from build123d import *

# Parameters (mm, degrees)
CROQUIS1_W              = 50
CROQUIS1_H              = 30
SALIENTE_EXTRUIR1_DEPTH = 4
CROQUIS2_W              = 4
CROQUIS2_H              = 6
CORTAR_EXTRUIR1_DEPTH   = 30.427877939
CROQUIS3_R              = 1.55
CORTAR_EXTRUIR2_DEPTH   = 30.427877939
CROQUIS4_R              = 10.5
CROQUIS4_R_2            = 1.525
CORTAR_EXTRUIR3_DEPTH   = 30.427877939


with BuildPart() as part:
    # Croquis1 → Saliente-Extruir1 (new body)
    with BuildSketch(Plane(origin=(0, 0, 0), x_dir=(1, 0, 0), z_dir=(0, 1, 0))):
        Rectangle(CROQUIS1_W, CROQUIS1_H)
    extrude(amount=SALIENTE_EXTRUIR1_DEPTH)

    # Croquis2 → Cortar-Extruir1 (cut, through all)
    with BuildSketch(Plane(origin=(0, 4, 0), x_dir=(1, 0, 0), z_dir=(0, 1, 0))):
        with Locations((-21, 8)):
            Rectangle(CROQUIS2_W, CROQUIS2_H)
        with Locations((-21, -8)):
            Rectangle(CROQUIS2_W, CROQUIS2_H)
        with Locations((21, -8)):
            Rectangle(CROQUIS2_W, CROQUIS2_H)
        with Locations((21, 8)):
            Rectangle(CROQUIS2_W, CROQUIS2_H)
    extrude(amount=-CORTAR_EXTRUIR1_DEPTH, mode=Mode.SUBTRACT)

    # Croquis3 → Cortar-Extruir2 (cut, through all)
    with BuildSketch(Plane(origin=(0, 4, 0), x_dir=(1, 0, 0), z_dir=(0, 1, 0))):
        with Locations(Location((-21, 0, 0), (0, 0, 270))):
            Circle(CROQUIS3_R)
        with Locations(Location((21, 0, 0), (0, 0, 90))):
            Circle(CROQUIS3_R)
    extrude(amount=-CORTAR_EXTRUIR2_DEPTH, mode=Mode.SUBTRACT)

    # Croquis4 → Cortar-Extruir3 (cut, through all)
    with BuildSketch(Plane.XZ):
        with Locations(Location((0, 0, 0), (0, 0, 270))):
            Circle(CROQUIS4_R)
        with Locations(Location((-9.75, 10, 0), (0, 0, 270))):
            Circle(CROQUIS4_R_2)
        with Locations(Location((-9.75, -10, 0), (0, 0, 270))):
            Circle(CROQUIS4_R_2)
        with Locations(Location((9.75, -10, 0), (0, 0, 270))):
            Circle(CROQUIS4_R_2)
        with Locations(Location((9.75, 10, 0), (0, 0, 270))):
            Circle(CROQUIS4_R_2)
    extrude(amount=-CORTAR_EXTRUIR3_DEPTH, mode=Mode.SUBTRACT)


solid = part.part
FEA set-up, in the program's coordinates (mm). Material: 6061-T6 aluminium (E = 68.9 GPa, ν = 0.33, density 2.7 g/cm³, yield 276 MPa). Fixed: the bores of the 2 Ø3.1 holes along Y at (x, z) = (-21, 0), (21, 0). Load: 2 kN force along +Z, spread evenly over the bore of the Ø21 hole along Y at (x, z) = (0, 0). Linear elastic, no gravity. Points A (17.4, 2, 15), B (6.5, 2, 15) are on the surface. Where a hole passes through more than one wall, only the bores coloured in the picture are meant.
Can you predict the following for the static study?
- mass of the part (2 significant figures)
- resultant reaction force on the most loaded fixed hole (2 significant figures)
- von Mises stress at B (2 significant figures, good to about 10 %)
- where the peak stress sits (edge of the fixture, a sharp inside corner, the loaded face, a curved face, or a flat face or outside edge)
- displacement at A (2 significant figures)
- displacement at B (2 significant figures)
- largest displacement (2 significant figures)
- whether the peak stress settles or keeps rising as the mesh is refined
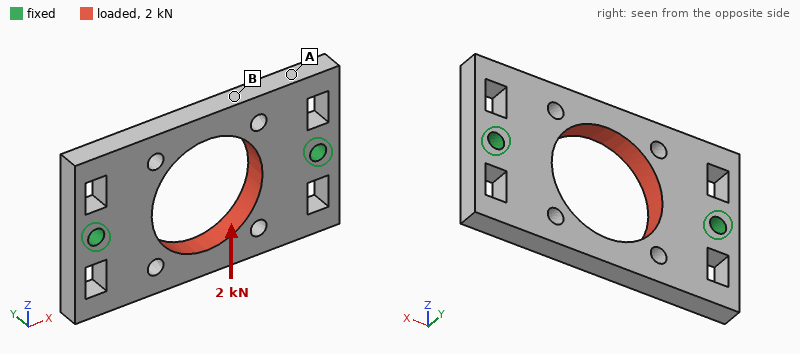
11 g
1.0 kN
29 MPa
edge of the fixture
6.9 µm
12 µm
15 µm
keeps rising
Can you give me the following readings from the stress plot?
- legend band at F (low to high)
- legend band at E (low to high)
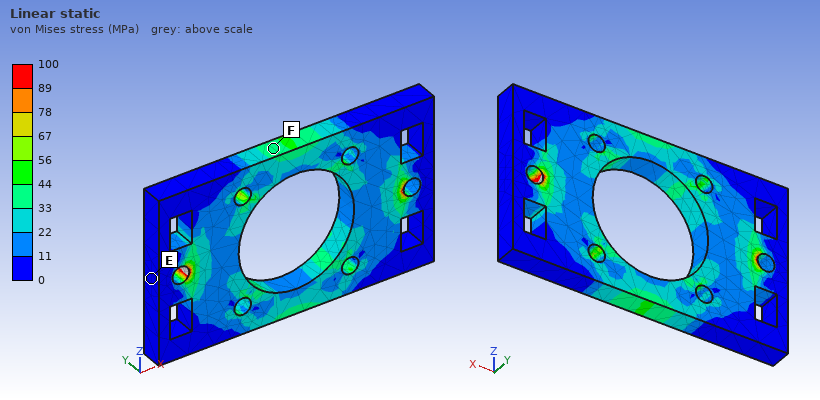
33 to 44 MPa
0 to 11 MPa
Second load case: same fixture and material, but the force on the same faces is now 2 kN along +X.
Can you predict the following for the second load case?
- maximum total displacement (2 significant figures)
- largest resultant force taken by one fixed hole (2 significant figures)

8.8 µm
1.0 kN
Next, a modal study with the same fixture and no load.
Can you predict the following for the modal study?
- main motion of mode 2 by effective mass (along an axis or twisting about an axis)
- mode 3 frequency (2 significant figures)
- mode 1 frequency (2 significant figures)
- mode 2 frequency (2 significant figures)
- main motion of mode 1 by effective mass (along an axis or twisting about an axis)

along Y
13 kHz
7100 Hz
8600 Hz
twisting about X
